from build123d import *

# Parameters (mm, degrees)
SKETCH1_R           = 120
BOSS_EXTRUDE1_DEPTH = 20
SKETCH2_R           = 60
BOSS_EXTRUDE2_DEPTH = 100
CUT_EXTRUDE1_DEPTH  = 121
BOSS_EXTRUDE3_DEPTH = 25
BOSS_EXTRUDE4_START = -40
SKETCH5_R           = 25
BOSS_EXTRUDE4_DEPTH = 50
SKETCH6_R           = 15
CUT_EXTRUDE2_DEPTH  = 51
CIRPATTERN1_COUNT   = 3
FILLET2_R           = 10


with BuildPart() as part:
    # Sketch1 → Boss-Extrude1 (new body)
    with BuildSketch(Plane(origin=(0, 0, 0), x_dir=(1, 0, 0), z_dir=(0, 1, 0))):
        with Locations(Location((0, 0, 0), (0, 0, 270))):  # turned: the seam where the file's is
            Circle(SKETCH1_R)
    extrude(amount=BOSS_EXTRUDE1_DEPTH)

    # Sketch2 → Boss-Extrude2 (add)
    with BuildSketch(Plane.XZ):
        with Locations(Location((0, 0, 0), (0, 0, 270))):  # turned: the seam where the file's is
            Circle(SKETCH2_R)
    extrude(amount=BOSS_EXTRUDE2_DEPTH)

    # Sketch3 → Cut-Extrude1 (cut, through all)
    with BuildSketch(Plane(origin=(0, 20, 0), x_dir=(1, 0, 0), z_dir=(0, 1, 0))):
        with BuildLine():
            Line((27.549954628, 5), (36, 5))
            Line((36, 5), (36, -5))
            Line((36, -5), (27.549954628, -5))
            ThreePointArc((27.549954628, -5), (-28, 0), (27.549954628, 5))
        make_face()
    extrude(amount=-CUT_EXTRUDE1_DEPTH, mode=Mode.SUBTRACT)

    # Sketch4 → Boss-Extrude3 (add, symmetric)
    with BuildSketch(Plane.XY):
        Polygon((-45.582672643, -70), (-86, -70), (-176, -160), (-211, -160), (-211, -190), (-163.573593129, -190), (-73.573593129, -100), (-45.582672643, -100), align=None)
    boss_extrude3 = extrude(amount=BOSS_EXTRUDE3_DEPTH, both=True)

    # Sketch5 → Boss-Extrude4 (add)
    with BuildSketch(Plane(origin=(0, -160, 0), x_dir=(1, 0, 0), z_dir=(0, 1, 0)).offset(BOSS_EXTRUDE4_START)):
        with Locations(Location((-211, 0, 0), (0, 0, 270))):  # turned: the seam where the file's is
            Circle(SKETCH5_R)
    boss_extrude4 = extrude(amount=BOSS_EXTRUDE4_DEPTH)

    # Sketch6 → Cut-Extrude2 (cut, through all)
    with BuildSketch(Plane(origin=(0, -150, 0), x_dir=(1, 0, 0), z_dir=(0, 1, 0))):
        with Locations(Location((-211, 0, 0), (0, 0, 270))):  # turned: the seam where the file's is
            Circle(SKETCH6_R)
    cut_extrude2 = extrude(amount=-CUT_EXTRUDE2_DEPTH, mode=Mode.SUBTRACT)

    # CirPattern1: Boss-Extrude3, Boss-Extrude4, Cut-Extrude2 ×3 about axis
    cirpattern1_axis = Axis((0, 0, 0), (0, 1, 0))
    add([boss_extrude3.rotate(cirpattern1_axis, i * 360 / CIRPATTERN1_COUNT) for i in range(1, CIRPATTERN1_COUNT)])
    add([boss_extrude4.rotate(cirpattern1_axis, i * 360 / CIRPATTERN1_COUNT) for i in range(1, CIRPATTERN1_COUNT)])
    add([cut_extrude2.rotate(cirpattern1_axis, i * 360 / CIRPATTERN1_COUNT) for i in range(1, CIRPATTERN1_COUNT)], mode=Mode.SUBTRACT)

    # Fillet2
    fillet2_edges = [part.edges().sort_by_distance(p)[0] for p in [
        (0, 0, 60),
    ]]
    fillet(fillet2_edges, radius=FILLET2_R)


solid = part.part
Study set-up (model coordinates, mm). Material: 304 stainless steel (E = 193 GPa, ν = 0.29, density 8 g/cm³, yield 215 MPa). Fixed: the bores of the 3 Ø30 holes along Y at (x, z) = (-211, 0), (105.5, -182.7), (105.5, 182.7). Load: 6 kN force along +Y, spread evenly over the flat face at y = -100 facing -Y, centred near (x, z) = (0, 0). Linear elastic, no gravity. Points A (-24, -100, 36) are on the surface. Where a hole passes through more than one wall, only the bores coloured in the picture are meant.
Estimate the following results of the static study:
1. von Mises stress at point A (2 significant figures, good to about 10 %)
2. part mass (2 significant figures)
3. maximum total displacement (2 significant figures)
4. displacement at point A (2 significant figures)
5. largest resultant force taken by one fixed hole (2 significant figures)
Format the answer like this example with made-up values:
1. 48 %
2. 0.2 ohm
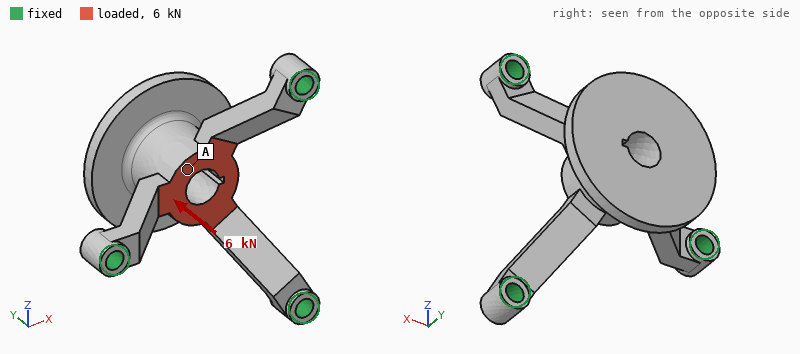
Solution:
1. 0.54 MPa
2. 22 kg
3. 4.5 µm
4. 4.4 µm
5. 3.0 kN
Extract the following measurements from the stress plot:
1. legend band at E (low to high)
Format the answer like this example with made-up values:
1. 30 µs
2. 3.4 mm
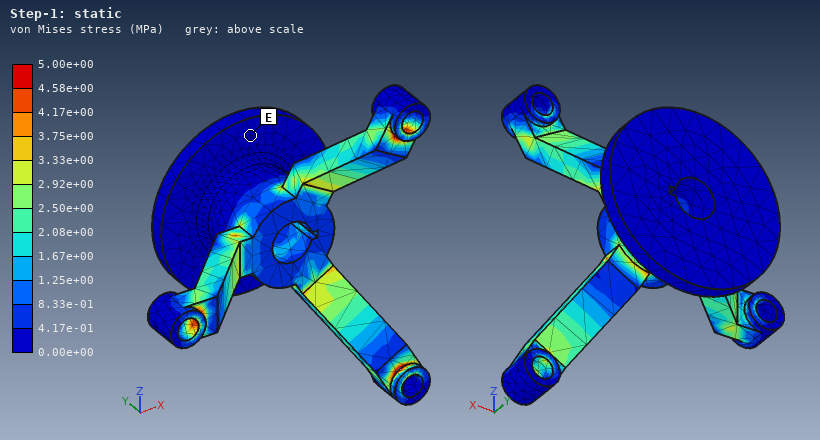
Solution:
1. 0.00e+00 to 4.17e-01 MPa
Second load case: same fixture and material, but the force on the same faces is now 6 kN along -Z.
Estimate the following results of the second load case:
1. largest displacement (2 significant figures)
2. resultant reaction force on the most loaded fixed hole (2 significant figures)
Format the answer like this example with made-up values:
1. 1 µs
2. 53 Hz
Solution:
1. 14 µm
2. 2.8 kN
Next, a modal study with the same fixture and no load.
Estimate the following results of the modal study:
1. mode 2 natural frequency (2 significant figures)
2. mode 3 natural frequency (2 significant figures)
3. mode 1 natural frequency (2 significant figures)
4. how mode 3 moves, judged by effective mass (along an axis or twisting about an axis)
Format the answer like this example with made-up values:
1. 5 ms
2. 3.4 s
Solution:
1. 920 Hz
2. 1100 Hz
3. 920 Hz
4. twisting about Y
